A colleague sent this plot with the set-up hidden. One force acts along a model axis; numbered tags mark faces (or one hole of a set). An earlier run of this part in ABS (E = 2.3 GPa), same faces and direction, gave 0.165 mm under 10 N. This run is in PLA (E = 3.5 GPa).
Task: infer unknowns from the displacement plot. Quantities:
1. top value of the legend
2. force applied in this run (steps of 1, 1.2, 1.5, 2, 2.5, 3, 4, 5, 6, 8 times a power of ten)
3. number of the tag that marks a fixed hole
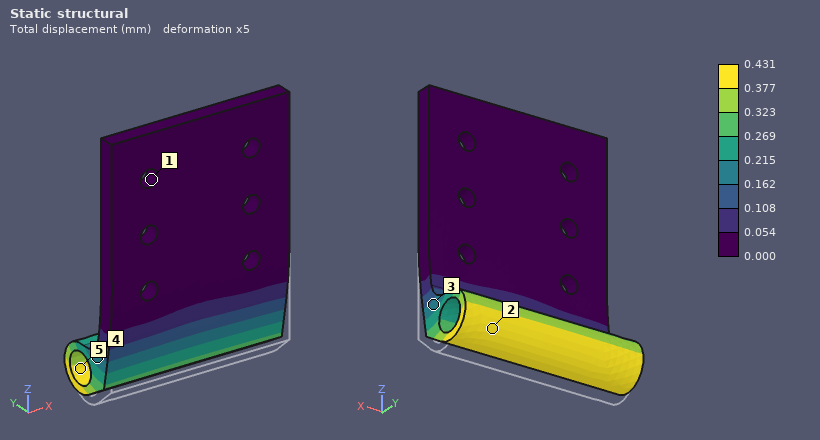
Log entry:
0.431 mm
40 N
1
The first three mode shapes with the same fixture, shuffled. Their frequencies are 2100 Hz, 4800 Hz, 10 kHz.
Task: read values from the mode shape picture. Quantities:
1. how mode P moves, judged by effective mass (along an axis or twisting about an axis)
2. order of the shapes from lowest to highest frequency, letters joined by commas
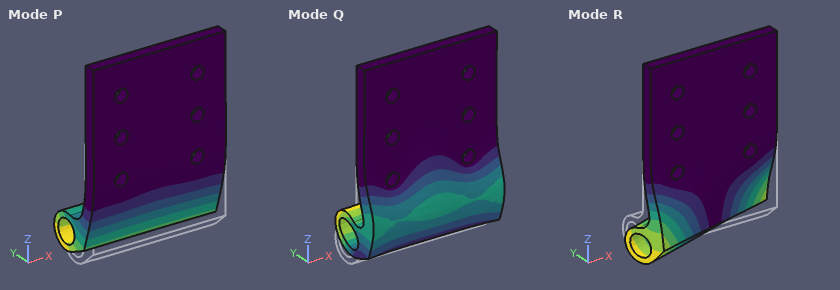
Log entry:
along Y
P, R, Q
